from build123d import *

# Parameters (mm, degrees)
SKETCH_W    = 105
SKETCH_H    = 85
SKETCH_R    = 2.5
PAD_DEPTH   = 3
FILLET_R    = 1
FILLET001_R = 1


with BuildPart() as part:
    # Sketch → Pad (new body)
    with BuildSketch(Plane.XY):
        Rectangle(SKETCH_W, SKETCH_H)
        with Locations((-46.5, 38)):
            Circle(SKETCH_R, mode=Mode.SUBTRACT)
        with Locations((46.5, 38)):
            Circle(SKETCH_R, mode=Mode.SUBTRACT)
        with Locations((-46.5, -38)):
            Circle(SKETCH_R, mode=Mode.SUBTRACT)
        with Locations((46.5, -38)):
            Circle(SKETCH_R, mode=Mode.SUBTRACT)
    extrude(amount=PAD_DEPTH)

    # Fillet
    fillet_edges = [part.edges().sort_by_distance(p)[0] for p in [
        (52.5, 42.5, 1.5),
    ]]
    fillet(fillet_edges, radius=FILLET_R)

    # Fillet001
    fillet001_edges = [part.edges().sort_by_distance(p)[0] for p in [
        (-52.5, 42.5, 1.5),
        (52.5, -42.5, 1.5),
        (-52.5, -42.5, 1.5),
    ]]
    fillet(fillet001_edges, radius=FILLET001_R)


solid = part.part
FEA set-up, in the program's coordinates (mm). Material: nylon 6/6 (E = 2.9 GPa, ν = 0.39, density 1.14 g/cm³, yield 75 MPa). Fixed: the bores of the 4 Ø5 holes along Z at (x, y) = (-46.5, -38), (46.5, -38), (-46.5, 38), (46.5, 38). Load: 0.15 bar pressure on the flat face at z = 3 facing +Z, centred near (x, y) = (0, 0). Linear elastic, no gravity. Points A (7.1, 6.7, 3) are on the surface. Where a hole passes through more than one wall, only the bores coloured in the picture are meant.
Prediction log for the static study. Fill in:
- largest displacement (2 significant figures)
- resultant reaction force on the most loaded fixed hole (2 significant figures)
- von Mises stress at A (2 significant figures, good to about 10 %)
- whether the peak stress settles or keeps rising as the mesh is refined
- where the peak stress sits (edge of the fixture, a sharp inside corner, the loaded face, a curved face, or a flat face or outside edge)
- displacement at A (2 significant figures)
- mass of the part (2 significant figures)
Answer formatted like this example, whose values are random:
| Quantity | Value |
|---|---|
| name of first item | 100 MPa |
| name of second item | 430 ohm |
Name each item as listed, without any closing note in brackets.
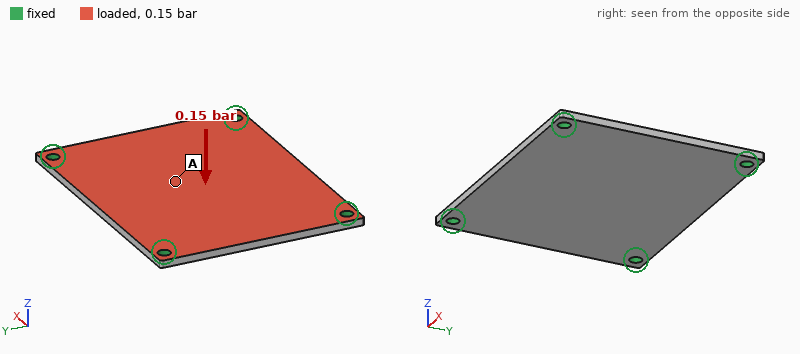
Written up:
| Quantity | Value |
|---|---|
| largest displacement | 0.81 mm |
| resultant reaction force on the most loaded fixed hole | 33 N |
| von Mises stress at A | 4.1 MPa |
| whether the peak stress settles or keeps rising as the mesh is refined | keeps rising |
| where the peak stress sits | edge of the fixture |
| displacement at A | 0.78 mm |
| mass of the part | 30 g |
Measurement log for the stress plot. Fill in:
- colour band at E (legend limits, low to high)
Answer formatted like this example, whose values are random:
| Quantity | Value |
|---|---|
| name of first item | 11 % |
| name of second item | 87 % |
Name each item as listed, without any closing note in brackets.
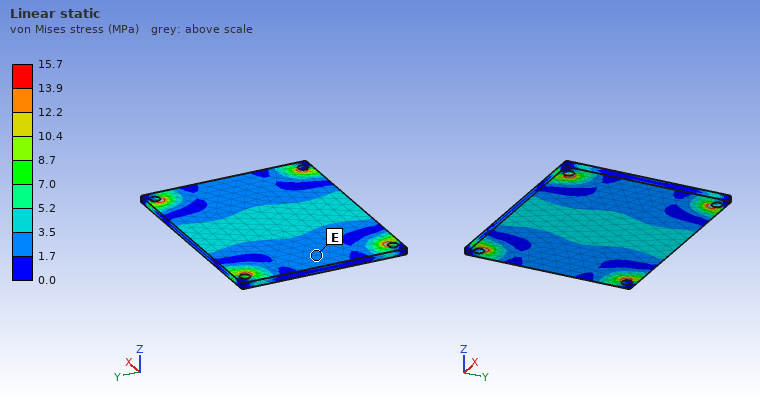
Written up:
| Quantity | Value |
|---|---|
| colour band at E | 1.7 to 3.5 MPa |
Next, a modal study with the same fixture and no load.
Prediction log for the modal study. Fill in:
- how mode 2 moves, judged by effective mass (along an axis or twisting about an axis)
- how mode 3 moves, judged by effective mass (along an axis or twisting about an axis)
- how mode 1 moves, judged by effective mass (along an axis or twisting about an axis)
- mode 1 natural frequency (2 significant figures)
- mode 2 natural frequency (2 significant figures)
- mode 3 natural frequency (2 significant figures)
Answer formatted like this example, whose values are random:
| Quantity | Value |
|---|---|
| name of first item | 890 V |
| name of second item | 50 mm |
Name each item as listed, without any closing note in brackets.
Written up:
| Quantity | Value |
|---|---|
| how mode 2 moves, judged by effective mass | twisting about X |
| how mode 3 moves, judged by effective mass | twisting about Y |
| how mode 1 moves, judged by effective mass | along Z |
| mode 1 natural frequency | 440 Hz |
| mode 2 natural frequency | 710 Hz |
| mode 3 natural frequency | 900 Hz |
